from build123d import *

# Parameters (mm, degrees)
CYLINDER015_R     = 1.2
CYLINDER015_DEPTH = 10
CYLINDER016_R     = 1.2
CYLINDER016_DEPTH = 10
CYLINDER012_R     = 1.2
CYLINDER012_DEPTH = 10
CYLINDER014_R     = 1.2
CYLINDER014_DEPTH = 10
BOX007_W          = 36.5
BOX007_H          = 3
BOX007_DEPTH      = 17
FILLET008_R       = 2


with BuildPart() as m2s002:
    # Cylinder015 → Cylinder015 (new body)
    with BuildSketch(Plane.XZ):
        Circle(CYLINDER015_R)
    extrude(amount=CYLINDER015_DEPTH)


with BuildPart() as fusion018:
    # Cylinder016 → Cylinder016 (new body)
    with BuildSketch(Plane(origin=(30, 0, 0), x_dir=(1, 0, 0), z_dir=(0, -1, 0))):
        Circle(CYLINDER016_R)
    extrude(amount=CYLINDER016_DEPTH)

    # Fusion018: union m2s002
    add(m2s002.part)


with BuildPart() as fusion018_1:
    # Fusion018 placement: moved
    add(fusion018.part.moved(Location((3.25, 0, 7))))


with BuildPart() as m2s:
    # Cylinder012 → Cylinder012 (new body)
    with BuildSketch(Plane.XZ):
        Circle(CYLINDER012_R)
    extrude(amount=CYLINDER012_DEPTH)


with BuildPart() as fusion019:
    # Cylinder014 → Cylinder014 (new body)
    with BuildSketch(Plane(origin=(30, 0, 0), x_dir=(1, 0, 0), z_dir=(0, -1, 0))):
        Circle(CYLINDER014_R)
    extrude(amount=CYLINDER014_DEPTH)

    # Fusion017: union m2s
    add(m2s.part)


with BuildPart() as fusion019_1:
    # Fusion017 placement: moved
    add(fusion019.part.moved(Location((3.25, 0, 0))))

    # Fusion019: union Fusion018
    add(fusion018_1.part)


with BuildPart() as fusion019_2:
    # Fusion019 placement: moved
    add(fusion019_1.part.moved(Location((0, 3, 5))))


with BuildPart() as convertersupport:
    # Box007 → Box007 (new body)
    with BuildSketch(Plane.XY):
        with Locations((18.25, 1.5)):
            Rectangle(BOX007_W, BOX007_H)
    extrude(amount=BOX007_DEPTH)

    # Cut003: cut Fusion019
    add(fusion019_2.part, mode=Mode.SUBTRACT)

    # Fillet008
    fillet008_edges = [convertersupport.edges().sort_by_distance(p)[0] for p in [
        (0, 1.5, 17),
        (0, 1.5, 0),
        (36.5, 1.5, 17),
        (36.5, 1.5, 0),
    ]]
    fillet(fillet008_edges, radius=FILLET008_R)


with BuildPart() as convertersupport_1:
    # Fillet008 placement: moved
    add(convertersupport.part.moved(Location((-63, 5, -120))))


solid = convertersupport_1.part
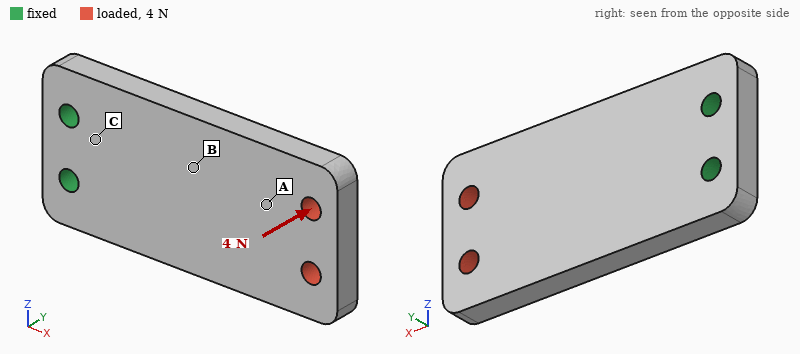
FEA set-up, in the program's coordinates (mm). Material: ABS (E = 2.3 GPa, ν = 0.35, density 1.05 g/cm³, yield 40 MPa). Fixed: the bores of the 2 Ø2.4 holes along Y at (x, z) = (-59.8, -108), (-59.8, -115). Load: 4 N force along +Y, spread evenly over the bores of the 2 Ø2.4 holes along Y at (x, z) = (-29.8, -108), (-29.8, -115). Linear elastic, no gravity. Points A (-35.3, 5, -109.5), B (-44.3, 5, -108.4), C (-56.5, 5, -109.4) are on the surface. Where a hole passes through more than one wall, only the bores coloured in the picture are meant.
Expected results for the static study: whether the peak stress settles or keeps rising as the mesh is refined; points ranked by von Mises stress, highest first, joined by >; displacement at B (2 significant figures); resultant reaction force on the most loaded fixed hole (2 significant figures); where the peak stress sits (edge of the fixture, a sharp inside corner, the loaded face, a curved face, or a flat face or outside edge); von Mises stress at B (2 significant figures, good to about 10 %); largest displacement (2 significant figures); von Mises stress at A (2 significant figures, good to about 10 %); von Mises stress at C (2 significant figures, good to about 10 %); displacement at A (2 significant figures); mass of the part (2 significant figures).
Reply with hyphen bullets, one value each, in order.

- keeps rising
- C > B > A
- 0.13 mm
- 2.0 N
- edge of the fixture
- 2.2 MPa
- 0.46 mm
- 0.96 MPa
- 4.1 MPa
- 0.28 mm
- 1.9 g
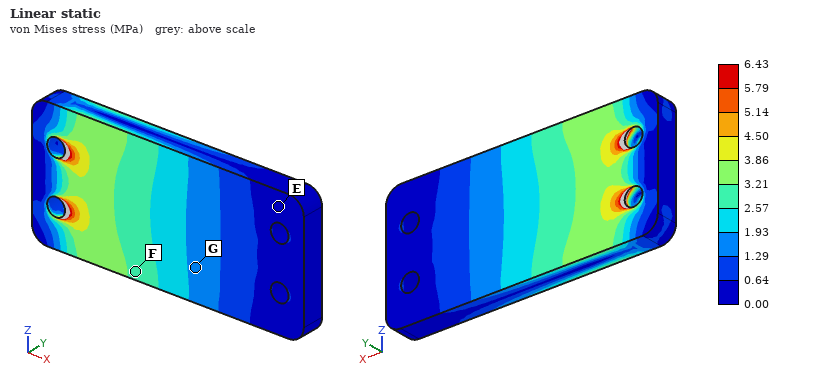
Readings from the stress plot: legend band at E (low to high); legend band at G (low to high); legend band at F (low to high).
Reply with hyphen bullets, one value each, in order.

- 0.00 to 0.64 MPa
- 1.29 to 1.93 MPa
- 2.57 to 3.21 MPa
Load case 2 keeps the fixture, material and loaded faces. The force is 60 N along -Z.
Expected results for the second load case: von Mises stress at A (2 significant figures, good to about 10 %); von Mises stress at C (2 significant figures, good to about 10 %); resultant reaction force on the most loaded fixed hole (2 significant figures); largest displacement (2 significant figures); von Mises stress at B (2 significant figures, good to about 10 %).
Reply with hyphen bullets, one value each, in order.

- 3.0 MPa
- 8.5 MPa
- 200 N
- 0.37 mm
- 3.5 MPa
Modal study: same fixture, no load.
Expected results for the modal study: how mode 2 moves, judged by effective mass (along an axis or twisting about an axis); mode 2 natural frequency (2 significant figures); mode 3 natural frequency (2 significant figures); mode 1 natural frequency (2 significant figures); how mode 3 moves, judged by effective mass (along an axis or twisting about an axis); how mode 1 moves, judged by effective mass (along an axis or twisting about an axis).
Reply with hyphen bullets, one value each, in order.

- twisting about X
- 2500 Hz
- 2700 Hz
- 690 Hz
- along Z
- along Y
